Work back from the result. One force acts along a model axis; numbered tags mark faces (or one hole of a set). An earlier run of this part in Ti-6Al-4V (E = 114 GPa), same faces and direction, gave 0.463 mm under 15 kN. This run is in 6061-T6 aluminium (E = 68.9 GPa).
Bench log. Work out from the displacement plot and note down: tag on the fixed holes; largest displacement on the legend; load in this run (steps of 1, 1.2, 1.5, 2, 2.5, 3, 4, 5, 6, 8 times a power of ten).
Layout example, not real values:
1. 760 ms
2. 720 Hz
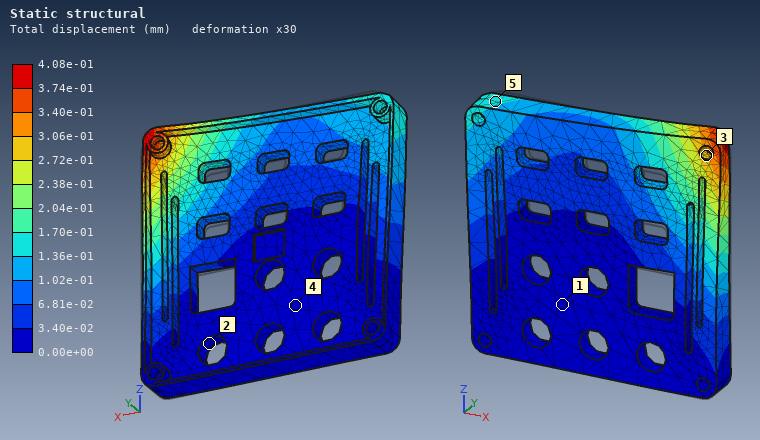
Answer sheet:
1. 2
2. 4.08e-01 mm
3. 8 kN
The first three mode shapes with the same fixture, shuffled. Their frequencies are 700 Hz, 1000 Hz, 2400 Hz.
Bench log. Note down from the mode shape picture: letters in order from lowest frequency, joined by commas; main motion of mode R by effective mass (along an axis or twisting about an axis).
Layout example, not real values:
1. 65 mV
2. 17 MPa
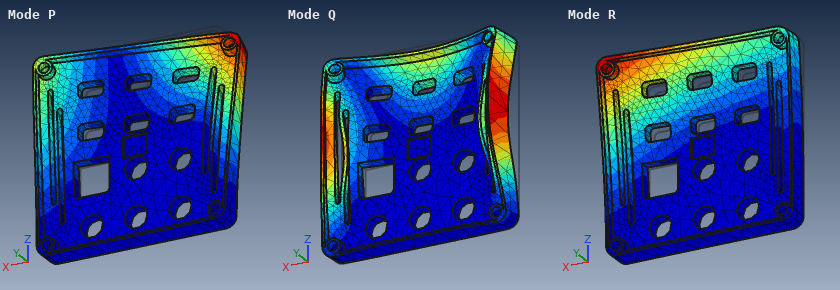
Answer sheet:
1. R, P, Q
2. along Y
